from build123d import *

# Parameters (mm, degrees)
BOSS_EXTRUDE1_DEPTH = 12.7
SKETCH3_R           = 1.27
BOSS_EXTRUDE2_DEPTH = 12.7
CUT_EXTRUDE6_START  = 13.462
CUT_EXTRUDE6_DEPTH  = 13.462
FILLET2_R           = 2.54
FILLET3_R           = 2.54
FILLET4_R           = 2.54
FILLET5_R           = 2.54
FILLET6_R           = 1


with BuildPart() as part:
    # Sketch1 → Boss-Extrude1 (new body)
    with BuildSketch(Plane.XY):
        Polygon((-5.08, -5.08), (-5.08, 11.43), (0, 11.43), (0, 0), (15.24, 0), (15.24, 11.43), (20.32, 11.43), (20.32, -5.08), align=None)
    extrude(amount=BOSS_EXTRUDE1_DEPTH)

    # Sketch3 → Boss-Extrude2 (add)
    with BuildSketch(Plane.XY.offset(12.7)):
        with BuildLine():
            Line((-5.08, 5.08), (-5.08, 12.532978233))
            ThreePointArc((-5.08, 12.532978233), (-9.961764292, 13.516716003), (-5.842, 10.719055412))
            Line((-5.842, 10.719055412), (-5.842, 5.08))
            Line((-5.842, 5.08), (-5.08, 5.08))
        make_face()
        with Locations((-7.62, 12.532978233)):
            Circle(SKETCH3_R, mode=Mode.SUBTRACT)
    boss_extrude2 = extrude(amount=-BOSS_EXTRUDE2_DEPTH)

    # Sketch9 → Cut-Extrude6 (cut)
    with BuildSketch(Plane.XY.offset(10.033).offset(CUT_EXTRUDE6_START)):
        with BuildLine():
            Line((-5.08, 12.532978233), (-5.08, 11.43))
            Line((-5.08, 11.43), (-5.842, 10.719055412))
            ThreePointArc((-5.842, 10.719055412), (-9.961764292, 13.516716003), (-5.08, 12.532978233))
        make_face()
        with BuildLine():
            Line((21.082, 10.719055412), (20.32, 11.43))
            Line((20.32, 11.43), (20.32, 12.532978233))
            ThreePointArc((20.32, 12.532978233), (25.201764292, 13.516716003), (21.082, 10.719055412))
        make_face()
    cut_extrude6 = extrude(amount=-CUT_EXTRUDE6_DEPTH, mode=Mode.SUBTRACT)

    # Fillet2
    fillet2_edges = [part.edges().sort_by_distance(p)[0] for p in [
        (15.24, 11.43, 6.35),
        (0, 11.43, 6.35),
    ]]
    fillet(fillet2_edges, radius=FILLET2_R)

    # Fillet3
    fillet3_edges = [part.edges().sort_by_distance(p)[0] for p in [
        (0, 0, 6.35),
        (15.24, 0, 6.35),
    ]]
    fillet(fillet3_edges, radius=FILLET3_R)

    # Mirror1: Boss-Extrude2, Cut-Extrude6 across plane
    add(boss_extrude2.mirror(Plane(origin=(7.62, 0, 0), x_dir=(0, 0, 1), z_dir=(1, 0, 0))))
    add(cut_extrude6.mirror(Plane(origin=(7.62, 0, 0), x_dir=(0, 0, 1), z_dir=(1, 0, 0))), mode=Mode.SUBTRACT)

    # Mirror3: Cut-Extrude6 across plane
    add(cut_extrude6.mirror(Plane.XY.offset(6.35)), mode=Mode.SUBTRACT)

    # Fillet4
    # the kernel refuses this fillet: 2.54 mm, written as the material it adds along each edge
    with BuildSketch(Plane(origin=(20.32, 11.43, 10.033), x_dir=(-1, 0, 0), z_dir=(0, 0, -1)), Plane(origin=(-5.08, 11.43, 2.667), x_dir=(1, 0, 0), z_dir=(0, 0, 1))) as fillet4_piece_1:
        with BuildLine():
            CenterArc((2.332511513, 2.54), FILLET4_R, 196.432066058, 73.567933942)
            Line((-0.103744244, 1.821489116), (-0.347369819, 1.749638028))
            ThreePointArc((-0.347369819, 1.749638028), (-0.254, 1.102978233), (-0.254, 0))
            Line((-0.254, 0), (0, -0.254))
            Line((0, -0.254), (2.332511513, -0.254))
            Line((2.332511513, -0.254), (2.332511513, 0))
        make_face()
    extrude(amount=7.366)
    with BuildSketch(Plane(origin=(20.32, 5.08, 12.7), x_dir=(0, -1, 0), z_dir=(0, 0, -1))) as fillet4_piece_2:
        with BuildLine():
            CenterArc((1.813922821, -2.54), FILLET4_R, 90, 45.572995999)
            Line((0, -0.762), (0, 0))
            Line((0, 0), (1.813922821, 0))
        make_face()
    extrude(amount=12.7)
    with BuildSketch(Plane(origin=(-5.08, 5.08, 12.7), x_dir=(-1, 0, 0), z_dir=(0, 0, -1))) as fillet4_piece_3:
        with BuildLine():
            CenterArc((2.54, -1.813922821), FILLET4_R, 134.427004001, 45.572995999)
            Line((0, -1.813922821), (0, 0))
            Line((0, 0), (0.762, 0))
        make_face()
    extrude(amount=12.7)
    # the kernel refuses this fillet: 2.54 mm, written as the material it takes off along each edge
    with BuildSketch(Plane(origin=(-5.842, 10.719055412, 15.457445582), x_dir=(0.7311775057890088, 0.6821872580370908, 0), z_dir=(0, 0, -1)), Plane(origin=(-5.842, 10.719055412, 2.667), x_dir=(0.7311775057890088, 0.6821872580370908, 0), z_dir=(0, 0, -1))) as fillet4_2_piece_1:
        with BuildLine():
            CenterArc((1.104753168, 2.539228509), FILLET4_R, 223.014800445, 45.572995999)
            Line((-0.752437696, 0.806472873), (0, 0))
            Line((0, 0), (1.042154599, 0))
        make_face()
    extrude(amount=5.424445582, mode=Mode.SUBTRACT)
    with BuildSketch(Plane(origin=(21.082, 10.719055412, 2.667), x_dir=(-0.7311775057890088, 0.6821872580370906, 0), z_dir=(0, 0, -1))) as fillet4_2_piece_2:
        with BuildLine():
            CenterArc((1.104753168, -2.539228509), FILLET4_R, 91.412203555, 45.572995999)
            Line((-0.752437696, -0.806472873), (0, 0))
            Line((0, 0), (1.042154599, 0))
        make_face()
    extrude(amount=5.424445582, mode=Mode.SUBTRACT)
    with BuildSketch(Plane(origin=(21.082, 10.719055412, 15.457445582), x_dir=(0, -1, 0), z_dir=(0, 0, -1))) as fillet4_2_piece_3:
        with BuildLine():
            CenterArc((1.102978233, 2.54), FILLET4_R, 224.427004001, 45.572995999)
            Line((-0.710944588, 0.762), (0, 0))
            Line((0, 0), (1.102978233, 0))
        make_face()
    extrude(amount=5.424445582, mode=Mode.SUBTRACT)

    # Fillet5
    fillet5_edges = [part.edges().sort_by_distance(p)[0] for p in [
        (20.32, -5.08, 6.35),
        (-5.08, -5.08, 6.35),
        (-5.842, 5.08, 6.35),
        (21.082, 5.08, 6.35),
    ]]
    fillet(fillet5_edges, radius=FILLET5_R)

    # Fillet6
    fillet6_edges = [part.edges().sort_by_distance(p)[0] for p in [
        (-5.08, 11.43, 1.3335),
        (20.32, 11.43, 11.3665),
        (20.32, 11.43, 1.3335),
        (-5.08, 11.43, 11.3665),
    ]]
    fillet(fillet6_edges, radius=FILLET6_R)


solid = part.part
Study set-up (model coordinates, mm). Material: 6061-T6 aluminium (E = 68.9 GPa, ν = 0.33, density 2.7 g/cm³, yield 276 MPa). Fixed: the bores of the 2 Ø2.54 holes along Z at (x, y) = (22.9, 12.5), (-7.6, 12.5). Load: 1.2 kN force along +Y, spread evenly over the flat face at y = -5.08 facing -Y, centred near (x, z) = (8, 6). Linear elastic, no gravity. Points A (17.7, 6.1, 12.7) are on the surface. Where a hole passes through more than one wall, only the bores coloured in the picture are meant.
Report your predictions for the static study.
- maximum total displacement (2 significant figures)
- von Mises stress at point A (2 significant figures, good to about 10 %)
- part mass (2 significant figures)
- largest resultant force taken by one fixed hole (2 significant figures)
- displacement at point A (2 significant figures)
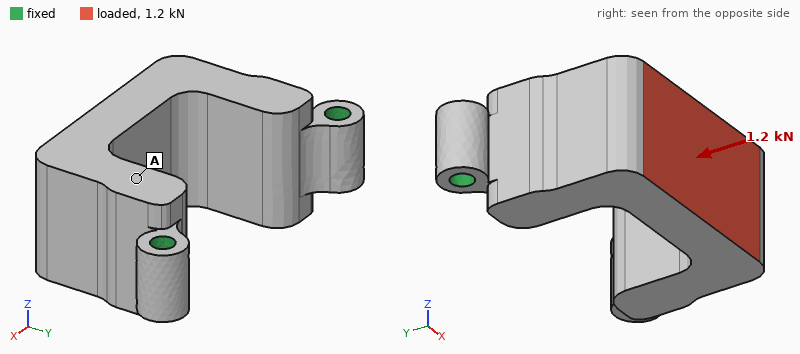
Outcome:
8.6 µm
11 MPa
9.3 g
660 N
3.6 µm
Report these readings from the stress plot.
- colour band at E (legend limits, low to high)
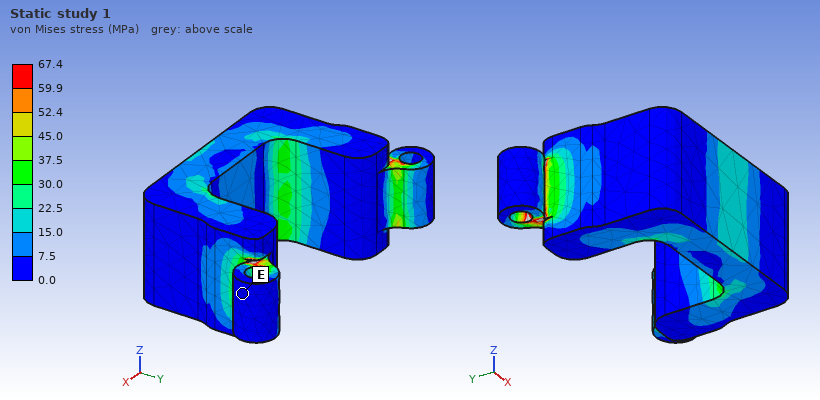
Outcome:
0.0 to 7.5 MPa
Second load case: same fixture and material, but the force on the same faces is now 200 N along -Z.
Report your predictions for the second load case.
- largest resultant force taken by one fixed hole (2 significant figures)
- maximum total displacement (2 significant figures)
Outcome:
100 N
31 µm
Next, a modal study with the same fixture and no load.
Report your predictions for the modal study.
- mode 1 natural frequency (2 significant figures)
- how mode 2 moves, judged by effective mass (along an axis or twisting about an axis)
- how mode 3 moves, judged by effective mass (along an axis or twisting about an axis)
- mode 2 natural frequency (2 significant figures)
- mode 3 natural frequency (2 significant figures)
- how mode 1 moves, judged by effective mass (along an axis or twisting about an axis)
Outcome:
6400 Hz
along X
twisting about Y
12 kHz
14 kHz
along Z
